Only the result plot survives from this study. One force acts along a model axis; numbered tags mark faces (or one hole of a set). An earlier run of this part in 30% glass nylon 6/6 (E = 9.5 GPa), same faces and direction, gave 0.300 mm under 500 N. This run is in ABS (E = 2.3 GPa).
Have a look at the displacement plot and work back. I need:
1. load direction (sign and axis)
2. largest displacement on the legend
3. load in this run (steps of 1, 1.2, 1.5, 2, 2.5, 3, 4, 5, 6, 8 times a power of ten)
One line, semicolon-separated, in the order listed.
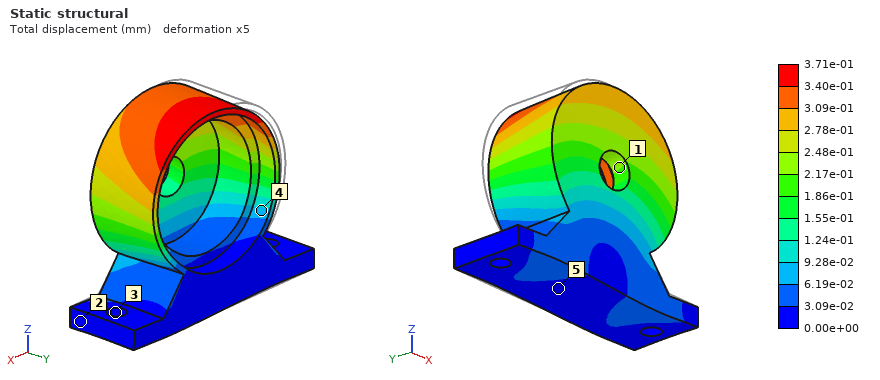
+X; 3.71e-01 mm; 150 N
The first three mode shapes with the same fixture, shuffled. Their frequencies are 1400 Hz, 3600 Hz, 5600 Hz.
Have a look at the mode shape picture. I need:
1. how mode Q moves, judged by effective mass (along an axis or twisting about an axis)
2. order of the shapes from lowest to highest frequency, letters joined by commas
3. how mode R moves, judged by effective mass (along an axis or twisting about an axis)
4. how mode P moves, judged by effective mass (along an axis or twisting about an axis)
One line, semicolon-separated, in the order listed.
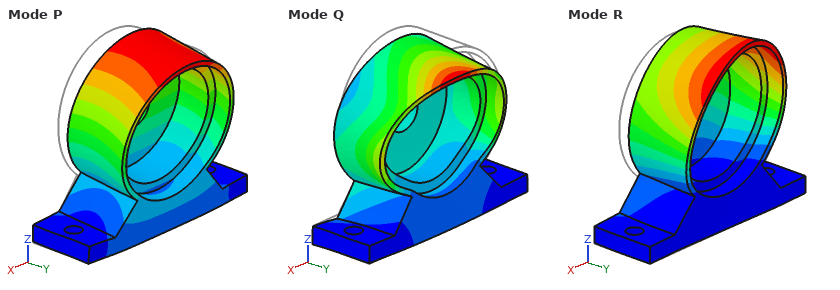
along Z; P, R, Q; along X; along Y
